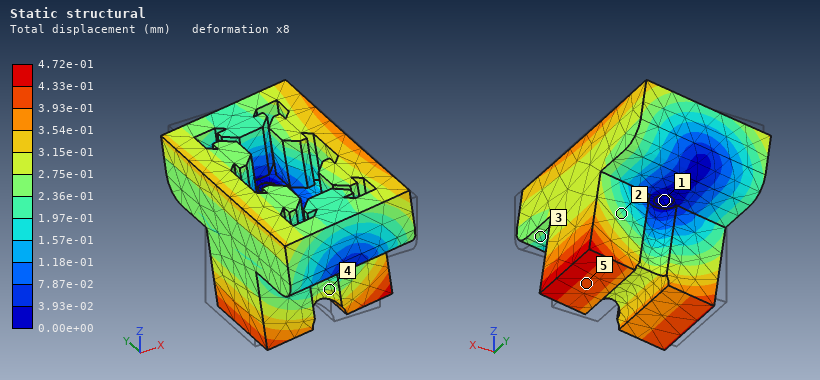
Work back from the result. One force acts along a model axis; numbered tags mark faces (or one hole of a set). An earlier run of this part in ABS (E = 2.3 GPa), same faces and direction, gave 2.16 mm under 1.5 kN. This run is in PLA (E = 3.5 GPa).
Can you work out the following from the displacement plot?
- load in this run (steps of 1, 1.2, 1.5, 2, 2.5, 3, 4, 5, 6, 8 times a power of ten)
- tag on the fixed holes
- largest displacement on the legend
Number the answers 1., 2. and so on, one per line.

1. 500 N
2. 1
3. 4.72e-01 mm
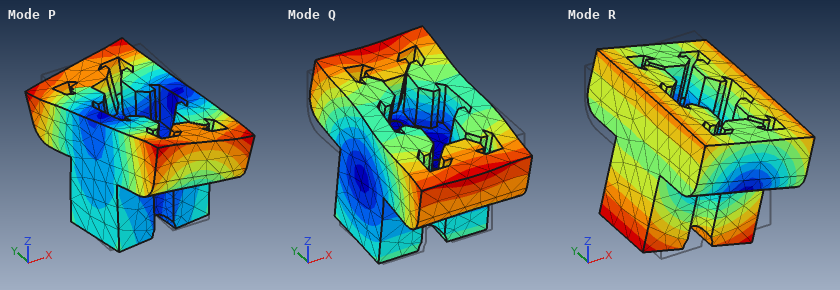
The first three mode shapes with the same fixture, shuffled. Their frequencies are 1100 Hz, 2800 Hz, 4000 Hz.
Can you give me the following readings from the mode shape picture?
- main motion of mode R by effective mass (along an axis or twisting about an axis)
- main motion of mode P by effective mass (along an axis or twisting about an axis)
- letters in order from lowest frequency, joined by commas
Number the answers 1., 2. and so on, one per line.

1. twisting about Y
2. twisting about Z
3. R, Q, P
